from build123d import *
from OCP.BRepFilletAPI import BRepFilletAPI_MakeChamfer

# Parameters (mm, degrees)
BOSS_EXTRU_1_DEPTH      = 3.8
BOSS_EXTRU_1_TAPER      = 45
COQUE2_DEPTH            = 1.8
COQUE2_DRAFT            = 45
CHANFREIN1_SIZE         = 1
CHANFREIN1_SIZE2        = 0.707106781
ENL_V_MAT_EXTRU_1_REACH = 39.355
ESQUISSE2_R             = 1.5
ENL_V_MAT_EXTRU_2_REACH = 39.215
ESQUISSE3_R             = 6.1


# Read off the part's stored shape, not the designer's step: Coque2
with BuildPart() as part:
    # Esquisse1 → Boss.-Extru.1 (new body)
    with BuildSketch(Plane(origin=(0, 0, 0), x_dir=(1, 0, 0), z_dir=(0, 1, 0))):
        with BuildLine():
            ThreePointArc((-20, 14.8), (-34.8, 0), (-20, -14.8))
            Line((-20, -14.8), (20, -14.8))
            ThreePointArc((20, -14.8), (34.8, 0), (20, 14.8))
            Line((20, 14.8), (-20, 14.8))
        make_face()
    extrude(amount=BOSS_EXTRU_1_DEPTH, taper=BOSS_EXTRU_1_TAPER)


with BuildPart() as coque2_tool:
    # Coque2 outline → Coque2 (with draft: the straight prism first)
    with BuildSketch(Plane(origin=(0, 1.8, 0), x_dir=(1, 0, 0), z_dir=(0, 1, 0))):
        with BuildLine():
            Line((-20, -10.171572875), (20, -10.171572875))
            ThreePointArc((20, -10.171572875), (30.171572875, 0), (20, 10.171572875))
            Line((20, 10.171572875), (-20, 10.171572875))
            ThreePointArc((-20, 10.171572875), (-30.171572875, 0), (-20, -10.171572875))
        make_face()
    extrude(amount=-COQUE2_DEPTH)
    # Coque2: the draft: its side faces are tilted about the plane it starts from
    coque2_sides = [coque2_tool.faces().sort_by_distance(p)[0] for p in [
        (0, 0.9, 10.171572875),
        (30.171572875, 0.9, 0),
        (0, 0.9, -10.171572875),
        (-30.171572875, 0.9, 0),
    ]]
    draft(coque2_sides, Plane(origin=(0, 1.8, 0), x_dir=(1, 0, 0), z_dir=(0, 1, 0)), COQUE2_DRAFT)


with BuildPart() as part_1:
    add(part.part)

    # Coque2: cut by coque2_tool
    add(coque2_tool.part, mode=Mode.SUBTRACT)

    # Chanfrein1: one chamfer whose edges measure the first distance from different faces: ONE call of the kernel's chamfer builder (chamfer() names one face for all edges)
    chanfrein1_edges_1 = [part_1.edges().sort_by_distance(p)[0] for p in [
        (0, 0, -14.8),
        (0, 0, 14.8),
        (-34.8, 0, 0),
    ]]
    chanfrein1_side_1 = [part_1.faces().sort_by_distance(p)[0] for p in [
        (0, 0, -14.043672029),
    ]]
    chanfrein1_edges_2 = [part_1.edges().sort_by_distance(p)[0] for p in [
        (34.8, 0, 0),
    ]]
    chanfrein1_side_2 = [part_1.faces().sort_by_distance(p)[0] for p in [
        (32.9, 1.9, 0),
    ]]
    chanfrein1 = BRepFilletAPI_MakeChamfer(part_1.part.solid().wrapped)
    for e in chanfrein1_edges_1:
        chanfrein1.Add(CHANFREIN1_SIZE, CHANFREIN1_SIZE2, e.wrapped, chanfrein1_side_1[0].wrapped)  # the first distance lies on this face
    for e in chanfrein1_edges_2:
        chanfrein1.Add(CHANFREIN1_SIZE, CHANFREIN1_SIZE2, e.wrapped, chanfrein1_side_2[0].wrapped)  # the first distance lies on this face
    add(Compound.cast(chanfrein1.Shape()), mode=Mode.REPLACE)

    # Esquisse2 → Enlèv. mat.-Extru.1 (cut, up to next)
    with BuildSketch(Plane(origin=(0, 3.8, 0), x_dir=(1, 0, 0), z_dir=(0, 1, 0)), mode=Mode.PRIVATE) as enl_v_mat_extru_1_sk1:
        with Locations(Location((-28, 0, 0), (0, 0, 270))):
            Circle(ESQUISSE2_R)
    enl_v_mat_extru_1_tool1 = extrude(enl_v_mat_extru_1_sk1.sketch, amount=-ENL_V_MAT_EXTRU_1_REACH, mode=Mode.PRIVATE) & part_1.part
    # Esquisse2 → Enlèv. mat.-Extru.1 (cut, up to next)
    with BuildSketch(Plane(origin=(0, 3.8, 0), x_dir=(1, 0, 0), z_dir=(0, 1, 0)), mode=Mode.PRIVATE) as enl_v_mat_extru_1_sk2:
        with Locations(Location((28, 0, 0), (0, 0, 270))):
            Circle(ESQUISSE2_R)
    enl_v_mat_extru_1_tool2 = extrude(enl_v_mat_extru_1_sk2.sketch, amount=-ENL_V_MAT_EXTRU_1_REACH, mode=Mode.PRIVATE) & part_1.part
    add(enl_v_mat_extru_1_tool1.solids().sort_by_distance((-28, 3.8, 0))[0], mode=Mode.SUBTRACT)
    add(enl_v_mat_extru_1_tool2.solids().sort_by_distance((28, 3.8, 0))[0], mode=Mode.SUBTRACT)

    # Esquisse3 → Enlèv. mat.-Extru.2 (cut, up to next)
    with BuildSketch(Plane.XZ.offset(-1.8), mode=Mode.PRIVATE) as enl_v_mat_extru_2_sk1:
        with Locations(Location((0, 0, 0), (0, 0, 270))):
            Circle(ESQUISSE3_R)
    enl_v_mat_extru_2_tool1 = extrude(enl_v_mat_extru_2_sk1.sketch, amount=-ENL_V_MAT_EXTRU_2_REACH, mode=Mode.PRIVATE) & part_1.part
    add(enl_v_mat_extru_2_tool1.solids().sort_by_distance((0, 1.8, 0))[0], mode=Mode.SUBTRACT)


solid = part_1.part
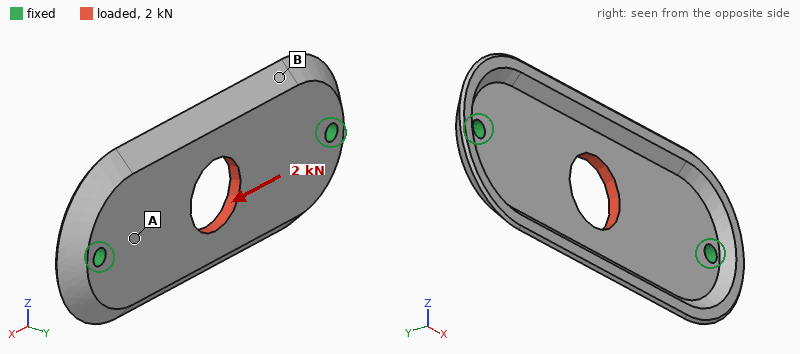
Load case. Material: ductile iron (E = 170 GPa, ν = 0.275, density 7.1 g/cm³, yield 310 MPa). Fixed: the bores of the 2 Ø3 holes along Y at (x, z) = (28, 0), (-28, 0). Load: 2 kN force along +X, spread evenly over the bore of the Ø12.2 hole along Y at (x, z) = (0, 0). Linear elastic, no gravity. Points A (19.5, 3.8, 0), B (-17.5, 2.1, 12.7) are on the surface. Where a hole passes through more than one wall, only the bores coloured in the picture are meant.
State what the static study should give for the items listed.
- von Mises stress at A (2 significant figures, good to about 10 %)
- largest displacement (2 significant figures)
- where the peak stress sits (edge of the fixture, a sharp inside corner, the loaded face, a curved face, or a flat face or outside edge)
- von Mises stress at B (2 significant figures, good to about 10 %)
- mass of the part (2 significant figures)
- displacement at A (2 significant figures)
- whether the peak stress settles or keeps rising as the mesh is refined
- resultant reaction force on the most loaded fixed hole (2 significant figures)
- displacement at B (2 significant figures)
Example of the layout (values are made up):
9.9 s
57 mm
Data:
37 MPa
5.0 µm
edge of the fixture
8.1 MPa
24 g
2.1 µm
keeps rising
1.0 kN
3.1 µm
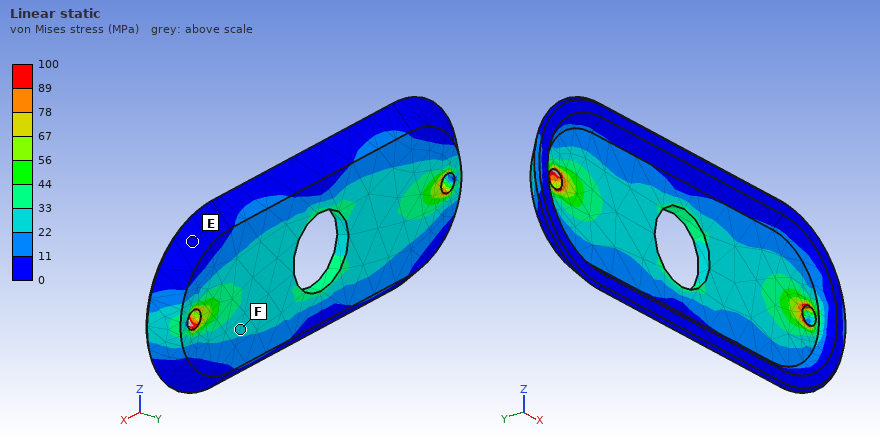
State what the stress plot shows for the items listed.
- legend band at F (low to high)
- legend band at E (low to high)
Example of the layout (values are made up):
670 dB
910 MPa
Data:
22 to 33 MPa
0 to 11 MPa
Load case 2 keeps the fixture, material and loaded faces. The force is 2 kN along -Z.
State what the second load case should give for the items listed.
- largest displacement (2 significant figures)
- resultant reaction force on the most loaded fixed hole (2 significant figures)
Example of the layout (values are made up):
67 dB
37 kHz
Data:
35 µm
1.0 kN
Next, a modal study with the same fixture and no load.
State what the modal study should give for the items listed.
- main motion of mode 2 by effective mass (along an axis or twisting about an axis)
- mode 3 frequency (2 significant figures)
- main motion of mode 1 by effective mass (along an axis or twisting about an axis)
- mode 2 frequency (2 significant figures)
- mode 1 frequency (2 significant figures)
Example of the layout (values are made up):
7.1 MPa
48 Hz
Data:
twisting about X
8200 Hz
along Y
4000 Hz
3600 Hz
